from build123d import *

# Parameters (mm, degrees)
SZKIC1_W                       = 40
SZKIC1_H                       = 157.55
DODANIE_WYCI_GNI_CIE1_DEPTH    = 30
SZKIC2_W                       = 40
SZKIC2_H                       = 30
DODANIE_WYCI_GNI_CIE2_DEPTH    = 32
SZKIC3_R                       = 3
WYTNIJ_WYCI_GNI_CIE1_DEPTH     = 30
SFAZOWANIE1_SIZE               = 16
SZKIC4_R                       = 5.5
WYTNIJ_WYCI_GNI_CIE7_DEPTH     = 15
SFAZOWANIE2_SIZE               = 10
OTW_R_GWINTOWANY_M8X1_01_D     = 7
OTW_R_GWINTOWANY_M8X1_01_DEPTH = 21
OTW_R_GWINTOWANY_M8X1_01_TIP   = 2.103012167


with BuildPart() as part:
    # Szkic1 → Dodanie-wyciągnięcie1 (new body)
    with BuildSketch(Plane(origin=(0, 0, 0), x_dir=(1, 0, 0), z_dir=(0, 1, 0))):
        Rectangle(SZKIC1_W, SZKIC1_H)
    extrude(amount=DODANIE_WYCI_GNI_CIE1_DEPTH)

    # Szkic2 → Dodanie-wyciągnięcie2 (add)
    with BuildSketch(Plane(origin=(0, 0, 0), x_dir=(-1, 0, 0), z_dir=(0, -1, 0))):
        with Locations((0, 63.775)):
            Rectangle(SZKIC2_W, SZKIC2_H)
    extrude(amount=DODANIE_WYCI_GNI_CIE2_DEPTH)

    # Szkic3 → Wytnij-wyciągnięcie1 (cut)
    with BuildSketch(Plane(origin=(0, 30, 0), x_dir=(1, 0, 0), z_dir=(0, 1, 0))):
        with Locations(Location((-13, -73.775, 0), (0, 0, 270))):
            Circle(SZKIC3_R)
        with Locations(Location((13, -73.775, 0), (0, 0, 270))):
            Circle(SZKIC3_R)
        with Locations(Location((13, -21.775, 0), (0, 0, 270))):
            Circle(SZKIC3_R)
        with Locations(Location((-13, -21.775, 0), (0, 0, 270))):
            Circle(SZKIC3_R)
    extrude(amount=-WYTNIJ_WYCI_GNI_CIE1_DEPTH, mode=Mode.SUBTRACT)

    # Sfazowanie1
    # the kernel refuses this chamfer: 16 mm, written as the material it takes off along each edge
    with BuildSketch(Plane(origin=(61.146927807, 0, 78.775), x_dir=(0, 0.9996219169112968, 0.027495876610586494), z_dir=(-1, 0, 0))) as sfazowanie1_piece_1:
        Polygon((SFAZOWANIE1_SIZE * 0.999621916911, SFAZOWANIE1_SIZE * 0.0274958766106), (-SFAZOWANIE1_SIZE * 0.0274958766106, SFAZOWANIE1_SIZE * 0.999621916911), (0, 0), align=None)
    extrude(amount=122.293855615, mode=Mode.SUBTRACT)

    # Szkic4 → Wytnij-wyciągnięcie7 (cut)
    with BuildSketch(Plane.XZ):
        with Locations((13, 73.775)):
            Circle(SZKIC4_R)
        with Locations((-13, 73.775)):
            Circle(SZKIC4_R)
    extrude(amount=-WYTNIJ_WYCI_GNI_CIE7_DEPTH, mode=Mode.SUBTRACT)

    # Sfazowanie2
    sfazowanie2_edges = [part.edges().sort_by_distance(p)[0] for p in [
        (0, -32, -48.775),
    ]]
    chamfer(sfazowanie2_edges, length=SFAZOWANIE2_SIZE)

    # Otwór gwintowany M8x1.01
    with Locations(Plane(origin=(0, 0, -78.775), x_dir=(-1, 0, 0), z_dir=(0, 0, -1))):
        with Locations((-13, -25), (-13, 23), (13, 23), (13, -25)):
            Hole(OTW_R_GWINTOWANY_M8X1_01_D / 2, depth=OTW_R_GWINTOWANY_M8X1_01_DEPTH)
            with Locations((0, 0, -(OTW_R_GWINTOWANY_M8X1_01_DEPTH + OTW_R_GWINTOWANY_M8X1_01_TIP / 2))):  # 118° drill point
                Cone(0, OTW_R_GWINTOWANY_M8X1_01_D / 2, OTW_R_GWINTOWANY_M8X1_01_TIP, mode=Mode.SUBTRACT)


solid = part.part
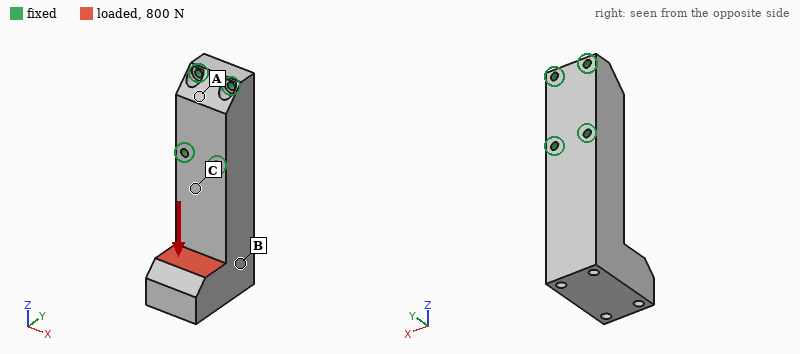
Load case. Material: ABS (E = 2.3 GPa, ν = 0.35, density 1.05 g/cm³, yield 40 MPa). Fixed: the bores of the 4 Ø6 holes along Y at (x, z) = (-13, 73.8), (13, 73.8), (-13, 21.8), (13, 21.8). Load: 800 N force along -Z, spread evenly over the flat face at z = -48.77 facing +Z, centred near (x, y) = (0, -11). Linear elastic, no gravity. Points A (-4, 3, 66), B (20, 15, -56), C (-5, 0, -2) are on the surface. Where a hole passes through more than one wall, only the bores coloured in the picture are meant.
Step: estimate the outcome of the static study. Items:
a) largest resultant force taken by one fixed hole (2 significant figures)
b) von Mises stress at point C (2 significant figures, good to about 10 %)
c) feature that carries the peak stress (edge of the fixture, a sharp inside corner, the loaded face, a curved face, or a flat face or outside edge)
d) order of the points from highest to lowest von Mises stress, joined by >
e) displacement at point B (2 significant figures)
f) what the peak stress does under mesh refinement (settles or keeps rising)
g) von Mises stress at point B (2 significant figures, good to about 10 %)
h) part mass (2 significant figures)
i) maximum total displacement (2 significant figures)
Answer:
390 N
4.1 MPa
edge of the fixture
C > B > A
0.31 mm
keeps rising
1.5 MPa
220 g
0.66 mm
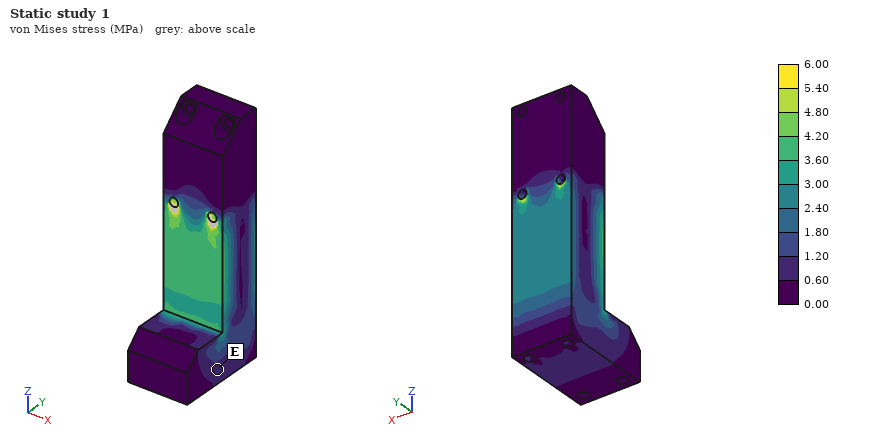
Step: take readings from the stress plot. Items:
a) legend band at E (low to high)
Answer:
0.60 to 1.20 MPa
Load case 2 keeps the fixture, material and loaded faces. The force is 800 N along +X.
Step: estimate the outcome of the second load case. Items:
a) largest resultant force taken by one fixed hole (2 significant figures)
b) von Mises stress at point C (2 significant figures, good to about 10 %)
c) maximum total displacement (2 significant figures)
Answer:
2.0 kN
5.9 MPa
0.93 mm
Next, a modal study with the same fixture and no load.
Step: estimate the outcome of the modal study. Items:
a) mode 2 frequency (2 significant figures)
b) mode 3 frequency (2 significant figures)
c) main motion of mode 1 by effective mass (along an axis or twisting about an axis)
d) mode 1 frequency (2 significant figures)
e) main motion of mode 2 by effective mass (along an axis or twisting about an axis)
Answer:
620 Hz
1300 Hz
along Y
480 Hz
along X
